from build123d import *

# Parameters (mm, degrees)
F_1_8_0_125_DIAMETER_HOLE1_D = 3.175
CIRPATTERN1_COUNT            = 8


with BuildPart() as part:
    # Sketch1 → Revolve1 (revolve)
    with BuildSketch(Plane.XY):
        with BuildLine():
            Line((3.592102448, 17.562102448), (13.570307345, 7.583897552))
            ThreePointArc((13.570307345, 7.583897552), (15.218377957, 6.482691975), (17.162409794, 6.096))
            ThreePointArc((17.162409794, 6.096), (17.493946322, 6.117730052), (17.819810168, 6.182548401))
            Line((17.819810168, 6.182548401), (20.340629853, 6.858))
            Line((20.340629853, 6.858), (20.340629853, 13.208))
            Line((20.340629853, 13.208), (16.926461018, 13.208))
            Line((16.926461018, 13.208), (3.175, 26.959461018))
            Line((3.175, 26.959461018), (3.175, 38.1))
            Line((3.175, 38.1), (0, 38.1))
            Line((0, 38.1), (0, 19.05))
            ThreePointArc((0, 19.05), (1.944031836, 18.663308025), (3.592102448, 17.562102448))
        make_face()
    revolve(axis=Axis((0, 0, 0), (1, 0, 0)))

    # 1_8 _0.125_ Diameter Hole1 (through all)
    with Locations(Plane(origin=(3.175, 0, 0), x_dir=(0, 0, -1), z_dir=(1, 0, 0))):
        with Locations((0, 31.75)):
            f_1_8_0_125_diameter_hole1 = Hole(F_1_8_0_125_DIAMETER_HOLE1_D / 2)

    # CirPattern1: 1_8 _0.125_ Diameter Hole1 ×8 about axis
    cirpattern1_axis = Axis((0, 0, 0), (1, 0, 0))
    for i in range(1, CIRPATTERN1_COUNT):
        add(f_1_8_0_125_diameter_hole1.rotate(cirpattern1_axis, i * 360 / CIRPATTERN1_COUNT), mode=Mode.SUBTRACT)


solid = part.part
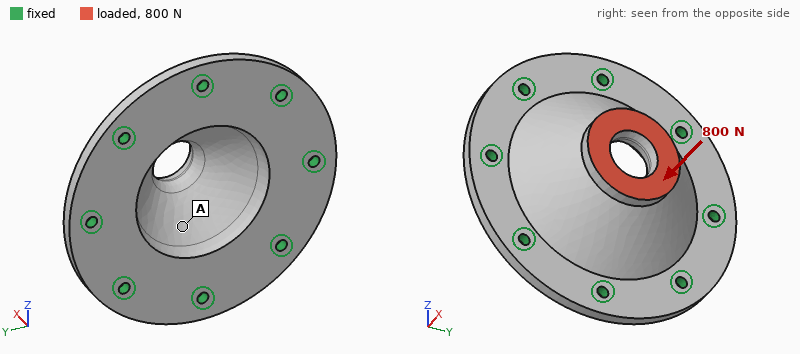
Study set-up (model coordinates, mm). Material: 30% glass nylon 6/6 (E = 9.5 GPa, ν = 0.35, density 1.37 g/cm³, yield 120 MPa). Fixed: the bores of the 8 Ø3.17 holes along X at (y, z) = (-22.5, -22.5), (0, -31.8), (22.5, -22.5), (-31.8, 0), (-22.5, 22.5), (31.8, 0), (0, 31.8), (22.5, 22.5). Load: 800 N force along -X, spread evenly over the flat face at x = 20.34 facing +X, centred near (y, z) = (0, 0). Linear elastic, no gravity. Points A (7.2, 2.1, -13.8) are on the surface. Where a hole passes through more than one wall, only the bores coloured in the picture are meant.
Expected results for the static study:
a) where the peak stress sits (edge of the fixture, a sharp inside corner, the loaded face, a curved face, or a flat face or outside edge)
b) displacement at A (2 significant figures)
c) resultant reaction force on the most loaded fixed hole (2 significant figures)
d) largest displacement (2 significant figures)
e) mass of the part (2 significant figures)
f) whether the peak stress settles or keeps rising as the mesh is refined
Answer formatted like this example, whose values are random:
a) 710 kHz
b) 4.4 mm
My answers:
a) edge of the fixture
b) 20 µm
c) 160 N
d) 23 µm
e) 33 g
f) keeps rising
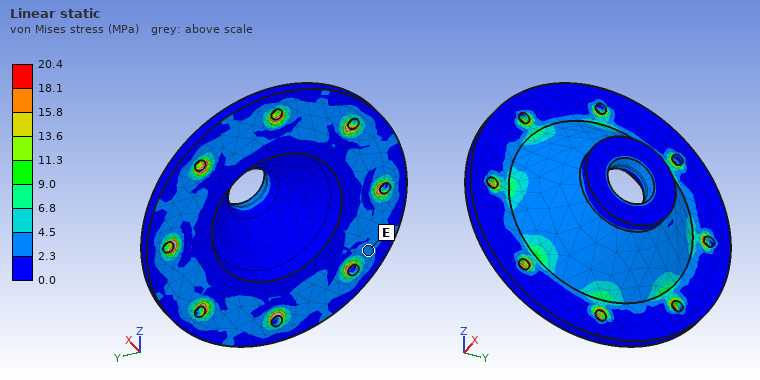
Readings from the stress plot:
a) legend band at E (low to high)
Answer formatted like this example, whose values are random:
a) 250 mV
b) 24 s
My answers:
a) 2.3 to 4.5 MPa
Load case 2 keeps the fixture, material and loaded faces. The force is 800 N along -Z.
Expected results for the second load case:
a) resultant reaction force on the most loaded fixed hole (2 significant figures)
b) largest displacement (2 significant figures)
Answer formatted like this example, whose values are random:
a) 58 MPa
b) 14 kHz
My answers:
a) 210 N
b) 28 µm
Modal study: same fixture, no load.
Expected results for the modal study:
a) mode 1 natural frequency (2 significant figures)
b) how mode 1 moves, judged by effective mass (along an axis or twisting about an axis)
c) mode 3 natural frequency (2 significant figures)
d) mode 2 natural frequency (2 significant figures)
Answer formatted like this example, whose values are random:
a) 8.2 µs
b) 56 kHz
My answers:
a) 6900 Hz
b) along X
c) 9100 Hz
d) 9100 Hz
